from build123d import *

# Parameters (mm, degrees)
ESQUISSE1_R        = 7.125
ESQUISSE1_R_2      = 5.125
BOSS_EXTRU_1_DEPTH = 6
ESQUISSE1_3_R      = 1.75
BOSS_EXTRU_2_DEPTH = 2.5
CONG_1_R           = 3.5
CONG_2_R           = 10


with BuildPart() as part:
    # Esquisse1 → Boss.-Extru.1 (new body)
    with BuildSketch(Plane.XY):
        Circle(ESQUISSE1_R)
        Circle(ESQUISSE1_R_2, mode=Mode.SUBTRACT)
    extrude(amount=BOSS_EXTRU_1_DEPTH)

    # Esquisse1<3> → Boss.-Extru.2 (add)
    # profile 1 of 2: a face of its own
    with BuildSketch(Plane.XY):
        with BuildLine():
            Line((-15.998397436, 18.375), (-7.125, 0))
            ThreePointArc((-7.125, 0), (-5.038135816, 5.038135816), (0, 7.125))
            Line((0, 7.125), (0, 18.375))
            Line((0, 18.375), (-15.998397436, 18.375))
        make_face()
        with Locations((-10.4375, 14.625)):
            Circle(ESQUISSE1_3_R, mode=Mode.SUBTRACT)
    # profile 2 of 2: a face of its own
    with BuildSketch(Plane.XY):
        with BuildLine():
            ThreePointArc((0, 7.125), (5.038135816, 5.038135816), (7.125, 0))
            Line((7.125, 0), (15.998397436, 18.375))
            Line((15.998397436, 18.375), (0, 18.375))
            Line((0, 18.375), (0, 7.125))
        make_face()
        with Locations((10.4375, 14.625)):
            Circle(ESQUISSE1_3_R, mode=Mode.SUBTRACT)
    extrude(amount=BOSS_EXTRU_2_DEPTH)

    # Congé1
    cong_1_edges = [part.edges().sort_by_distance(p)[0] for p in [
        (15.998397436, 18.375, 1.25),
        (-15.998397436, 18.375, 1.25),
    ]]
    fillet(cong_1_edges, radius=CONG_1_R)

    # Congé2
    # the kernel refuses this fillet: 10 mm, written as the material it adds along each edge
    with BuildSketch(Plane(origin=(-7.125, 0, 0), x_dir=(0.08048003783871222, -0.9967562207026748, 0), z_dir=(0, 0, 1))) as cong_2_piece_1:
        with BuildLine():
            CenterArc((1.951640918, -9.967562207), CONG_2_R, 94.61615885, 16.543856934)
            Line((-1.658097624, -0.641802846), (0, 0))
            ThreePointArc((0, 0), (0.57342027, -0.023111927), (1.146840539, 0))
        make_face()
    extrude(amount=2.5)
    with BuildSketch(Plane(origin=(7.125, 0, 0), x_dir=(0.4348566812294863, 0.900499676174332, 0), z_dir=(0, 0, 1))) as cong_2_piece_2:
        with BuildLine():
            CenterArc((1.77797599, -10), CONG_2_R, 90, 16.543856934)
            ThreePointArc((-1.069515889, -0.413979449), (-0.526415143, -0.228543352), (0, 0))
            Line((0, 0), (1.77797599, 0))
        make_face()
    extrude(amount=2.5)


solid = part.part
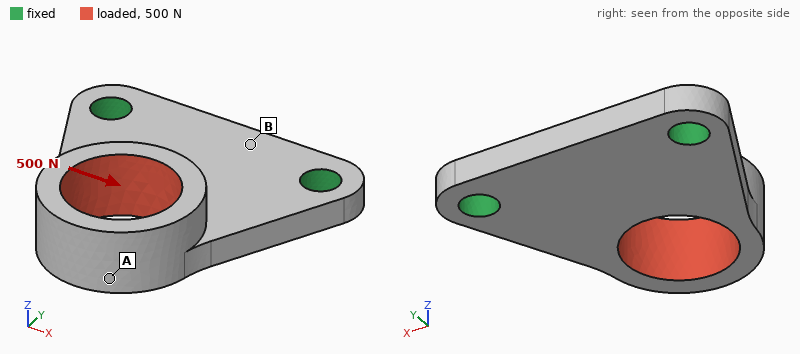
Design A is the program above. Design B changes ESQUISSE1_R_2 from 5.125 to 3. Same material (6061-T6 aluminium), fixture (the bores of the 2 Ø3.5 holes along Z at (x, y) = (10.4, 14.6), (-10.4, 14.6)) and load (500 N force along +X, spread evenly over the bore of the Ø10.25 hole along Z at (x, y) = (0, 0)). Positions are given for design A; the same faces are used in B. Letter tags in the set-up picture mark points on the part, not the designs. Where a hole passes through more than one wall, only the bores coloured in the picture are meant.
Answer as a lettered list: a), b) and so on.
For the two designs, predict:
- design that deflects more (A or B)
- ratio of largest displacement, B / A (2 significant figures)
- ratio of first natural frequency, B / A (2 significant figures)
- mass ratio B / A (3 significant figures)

a) A
b) 0.48
c) 0.83
d) 1.26
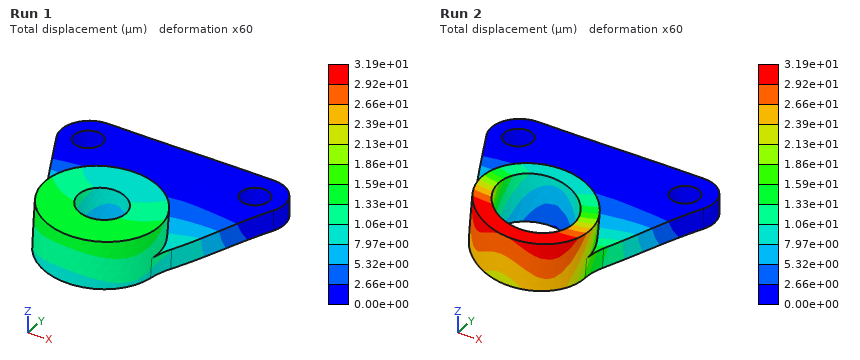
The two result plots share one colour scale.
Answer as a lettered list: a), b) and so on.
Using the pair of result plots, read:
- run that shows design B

a) Run 1
